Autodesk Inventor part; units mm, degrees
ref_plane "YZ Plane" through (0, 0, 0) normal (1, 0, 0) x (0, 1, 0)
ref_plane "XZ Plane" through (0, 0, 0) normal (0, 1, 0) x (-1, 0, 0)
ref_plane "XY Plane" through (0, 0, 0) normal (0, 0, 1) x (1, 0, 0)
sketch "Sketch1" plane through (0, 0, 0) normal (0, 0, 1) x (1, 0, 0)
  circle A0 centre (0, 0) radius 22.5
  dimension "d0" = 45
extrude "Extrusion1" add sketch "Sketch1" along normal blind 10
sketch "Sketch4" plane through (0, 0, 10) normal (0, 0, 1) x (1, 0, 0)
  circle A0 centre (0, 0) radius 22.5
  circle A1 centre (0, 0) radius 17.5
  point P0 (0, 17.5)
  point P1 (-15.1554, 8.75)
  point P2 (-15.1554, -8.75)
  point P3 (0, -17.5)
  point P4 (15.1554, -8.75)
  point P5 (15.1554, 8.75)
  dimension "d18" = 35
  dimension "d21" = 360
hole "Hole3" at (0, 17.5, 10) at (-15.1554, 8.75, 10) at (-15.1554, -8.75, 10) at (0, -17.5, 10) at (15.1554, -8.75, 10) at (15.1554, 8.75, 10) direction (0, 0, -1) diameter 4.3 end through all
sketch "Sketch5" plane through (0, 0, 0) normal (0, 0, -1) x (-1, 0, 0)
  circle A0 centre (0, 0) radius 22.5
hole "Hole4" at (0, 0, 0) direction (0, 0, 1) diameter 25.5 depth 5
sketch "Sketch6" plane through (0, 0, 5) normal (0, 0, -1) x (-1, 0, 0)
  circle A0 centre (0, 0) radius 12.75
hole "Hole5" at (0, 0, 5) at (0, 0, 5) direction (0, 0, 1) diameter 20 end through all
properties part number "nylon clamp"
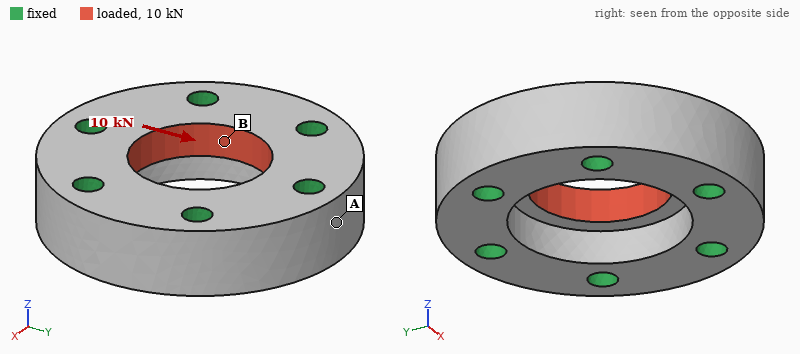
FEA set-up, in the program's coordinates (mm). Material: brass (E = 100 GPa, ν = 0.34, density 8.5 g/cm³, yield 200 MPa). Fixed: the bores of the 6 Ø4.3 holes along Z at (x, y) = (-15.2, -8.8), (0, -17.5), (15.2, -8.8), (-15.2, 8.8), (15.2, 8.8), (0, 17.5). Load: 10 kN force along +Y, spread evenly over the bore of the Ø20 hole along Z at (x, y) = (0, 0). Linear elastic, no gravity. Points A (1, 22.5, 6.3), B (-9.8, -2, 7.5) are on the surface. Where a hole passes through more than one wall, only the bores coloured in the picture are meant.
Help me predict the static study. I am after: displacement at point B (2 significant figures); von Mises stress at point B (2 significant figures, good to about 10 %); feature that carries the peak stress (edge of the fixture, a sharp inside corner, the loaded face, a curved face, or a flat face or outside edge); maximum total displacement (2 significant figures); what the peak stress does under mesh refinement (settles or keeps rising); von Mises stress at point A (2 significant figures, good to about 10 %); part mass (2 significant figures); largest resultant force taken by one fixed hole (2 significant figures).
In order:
2.9 µm
54 MPa
edge of the fixture
3.8 µm
keeps rising
7.9 MPa
93 g
2.2 kN
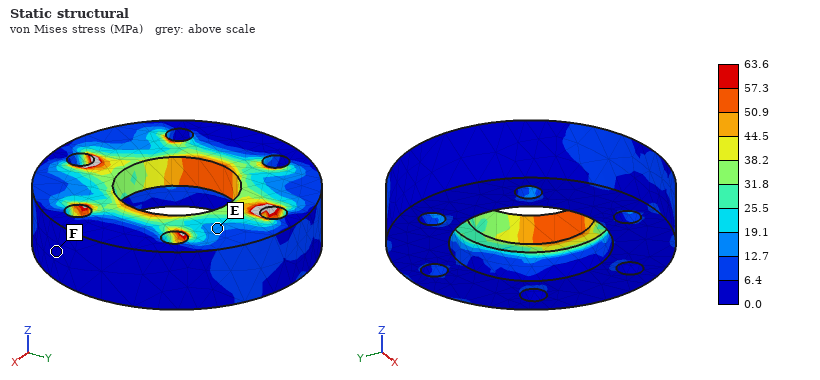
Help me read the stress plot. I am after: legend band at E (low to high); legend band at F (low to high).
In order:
12.7 to 19.1 MPa
0.0 to 6.4 MPa
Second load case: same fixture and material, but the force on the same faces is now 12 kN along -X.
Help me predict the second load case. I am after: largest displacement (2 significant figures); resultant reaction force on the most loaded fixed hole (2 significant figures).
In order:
4.9 µm
2.4 kN
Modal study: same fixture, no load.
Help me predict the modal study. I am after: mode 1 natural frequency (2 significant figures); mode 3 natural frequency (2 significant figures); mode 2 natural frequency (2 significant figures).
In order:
49 kHz
50 kHz
49 kHz
